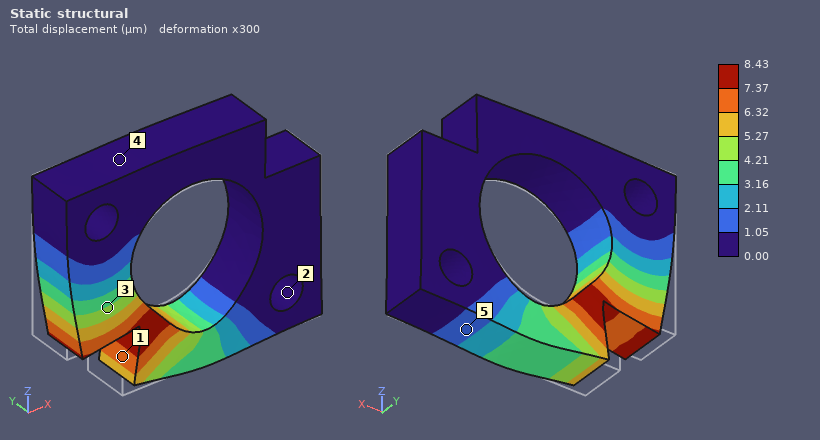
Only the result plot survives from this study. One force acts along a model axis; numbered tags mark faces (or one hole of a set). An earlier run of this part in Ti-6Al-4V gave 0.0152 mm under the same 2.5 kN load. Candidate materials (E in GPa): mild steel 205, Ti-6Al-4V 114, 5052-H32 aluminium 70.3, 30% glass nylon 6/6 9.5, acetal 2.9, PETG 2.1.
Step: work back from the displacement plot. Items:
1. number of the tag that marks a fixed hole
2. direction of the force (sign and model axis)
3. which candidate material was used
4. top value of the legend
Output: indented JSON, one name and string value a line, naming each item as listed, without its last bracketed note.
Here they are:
{
  "number of the tag that marks a fixed hole": "2",
  "direction of the force": "+X",
  "which candidate material was used": "mild steel",
  "top value of the legend": "8.43 µm"
}
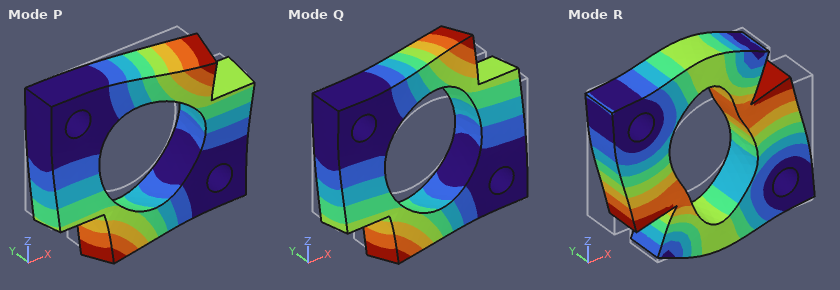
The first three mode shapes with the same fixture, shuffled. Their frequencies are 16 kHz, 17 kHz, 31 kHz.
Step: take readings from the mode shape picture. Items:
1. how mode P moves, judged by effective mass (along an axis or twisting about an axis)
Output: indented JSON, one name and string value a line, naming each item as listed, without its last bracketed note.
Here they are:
{
  "how mode P moves, judged by effective mass": "along Y"
}
